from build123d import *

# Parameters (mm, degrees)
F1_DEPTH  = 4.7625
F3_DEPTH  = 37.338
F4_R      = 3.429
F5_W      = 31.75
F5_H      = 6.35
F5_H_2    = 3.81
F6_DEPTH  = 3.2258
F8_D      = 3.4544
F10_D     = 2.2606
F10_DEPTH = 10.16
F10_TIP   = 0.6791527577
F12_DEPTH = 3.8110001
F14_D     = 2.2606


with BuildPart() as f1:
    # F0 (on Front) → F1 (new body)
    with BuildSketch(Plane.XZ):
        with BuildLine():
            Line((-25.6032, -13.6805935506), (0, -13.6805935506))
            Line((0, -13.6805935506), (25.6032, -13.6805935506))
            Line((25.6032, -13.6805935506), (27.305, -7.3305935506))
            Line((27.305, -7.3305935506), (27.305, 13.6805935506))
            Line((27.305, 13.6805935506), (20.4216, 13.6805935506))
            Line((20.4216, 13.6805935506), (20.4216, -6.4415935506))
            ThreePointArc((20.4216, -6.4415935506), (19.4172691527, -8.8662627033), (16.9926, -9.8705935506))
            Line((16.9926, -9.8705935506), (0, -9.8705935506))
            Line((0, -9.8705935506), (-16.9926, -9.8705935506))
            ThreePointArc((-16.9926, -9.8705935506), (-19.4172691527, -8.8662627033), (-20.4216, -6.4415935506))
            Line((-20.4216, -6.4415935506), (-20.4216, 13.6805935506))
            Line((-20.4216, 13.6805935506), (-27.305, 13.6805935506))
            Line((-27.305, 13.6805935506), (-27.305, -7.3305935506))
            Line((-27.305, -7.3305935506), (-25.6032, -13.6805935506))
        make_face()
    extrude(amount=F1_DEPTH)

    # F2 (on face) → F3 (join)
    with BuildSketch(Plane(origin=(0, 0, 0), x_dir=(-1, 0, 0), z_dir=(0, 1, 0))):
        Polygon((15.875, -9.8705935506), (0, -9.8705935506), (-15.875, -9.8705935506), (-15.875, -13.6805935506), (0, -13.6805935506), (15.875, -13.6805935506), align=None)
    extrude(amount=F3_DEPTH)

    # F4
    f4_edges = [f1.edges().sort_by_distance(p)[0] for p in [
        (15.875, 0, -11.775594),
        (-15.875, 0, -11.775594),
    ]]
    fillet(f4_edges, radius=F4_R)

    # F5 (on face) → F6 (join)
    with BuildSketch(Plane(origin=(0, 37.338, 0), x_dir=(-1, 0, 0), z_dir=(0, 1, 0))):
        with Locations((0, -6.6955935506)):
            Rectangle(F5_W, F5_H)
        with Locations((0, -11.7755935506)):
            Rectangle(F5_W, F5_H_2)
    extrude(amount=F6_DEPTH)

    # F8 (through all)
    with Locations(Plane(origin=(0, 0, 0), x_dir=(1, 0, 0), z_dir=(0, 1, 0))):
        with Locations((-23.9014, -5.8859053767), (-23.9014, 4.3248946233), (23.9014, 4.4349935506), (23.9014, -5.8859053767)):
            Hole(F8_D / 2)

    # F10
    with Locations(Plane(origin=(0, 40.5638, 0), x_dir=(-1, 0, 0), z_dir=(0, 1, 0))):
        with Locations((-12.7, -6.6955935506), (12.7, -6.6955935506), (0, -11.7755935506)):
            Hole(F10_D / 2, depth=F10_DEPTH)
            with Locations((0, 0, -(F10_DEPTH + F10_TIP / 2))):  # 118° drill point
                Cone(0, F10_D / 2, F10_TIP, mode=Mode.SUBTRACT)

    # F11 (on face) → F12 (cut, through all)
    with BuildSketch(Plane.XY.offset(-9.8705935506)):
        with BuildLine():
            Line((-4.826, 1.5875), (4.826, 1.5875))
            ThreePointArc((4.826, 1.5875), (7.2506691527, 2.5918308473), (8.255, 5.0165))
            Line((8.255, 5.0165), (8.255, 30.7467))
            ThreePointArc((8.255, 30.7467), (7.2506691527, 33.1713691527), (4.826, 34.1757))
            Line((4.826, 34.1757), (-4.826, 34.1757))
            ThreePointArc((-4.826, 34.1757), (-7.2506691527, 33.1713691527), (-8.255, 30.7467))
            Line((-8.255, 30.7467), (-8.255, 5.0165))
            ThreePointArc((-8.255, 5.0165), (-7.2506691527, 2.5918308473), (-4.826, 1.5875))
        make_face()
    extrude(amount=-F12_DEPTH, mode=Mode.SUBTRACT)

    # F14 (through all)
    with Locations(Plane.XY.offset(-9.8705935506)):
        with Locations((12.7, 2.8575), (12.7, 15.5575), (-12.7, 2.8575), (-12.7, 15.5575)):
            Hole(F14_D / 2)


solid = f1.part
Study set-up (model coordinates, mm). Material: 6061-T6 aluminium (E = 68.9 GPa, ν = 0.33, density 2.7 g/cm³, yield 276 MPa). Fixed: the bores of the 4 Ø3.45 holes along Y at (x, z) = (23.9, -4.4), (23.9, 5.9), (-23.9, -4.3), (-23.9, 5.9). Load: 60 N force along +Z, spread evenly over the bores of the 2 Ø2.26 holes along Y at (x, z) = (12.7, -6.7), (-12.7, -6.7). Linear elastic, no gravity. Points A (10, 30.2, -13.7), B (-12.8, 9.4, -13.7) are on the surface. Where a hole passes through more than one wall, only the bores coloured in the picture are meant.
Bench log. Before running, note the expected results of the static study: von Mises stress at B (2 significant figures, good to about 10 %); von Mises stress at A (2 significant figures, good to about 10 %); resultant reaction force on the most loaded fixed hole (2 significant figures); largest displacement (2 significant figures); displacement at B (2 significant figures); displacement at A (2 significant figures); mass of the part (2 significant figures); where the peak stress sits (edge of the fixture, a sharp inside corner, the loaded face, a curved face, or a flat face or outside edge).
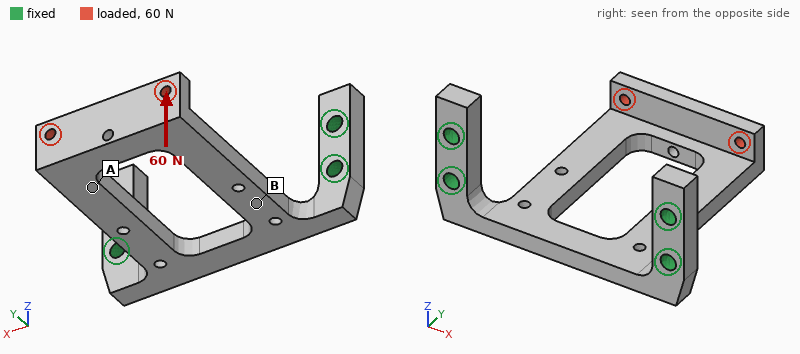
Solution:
47 MPa
15 MPa
47 N
0.60 mm
0.11 mm
0.41 mm
16 g
a curved face
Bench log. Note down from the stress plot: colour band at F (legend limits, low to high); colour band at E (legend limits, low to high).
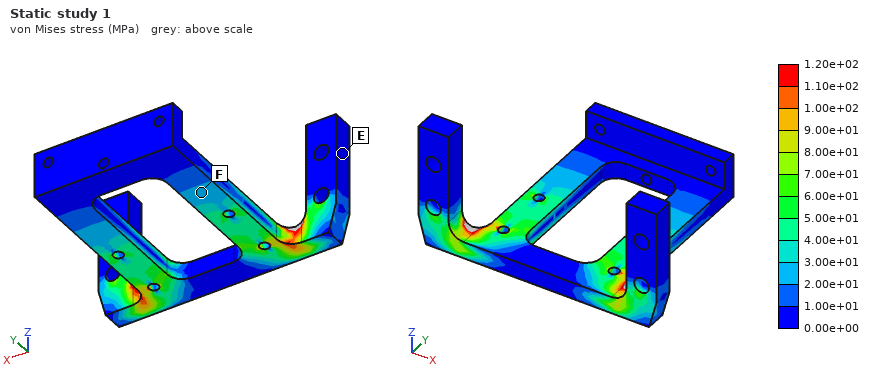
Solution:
2.00e+01 to 3.00e+01 MPa
0.00e+00 to 1.00e+01 MPa
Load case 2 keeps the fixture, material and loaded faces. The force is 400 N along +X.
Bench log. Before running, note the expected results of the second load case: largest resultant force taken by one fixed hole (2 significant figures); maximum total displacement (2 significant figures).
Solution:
470 N
0.33 mm
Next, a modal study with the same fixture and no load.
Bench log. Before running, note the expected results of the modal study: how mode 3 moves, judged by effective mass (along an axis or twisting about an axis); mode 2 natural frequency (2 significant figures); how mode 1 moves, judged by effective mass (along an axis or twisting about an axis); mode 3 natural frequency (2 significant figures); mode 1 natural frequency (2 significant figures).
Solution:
along X
2700 Hz
along Z
3600 Hz
760 Hz
